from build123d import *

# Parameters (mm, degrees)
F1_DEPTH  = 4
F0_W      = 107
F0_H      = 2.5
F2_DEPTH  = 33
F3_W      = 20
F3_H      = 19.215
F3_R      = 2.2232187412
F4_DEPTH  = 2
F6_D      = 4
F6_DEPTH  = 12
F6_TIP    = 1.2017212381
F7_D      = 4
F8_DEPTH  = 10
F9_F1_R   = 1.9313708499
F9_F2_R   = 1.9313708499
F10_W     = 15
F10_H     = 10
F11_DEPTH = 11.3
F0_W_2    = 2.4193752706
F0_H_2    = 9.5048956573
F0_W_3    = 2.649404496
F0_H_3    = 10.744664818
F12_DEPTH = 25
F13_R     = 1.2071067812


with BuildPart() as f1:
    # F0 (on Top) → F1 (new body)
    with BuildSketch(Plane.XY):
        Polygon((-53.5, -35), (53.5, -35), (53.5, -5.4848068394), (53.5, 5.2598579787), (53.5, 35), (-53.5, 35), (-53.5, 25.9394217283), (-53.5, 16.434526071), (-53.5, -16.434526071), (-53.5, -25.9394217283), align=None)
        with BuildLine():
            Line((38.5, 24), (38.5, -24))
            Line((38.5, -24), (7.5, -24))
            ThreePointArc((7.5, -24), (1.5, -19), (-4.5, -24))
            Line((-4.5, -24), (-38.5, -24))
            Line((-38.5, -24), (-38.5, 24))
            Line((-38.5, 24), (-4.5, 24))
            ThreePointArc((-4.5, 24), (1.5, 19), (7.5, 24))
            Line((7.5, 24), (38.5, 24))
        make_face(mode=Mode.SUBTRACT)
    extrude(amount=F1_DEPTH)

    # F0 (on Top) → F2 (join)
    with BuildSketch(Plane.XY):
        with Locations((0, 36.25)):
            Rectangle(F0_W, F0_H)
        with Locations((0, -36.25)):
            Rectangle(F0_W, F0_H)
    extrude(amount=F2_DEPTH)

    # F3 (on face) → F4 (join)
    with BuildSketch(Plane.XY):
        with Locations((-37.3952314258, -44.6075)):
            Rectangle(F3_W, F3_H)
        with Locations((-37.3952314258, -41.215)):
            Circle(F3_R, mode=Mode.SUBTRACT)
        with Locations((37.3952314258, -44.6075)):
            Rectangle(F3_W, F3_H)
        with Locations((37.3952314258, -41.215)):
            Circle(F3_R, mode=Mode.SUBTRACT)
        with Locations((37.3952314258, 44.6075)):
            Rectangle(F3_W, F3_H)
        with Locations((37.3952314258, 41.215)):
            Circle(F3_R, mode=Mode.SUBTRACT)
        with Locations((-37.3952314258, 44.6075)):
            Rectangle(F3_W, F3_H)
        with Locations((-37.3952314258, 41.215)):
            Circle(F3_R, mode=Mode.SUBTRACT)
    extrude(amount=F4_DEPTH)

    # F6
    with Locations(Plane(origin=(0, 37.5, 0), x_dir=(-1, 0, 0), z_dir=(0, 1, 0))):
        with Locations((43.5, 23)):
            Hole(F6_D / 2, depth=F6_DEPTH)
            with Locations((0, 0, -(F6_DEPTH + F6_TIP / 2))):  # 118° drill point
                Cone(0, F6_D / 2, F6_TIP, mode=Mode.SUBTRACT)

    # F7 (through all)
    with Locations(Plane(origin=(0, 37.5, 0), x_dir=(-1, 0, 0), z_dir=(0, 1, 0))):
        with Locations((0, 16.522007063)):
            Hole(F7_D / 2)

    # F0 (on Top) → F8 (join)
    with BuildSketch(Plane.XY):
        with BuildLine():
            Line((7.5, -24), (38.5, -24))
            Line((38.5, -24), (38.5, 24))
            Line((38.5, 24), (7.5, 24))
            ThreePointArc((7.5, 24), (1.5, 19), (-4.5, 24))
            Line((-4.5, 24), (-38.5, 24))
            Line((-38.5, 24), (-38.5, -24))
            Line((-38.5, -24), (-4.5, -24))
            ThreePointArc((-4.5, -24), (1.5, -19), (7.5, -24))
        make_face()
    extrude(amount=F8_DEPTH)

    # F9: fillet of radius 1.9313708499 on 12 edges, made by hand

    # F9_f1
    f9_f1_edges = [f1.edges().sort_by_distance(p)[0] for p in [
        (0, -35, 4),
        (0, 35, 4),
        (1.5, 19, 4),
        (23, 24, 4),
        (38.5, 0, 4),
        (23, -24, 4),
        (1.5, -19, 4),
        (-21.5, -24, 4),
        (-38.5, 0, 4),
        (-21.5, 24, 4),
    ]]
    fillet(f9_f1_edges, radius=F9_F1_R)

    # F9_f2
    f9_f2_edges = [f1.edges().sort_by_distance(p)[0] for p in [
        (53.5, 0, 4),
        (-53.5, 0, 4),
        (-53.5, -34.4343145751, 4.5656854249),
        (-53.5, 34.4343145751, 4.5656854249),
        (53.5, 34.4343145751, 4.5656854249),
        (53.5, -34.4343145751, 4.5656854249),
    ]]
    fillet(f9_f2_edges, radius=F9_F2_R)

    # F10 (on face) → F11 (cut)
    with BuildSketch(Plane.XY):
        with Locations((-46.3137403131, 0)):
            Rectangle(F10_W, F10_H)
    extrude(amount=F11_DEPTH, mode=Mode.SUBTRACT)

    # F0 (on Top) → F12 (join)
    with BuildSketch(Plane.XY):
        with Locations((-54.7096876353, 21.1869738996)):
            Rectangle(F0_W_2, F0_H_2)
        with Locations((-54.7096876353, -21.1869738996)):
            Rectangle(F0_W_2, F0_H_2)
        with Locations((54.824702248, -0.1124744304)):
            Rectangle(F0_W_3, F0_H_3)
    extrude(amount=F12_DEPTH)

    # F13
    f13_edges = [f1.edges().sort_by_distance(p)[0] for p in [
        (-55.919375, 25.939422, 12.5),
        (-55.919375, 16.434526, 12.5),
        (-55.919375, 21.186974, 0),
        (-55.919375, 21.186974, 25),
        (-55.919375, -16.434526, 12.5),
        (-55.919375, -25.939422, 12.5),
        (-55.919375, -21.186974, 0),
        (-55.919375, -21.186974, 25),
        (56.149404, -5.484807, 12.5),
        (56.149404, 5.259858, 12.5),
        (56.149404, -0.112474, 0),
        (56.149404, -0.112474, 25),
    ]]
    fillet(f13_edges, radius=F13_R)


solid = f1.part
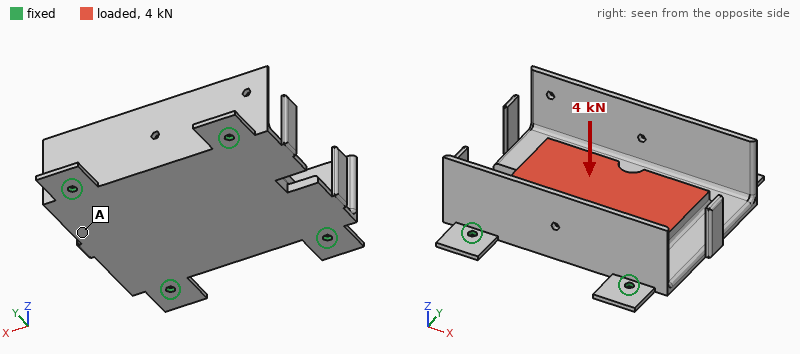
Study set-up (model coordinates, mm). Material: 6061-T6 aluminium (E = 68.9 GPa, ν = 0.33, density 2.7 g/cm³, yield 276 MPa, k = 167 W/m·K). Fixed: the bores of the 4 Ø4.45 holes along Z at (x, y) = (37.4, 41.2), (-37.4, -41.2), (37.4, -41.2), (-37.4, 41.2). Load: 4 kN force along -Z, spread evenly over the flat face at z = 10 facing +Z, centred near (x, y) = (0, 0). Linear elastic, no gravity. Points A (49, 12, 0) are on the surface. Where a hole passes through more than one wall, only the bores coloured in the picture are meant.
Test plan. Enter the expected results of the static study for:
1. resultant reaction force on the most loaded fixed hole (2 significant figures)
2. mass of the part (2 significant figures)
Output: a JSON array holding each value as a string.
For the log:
["1.9 kN", "200 g"]
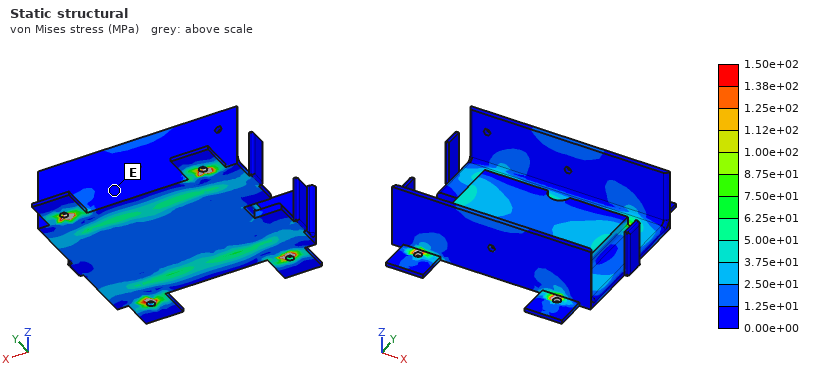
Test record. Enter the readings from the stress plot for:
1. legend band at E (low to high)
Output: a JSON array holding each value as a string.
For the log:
["0.00e+00 to 1.25e+01 MPa"]
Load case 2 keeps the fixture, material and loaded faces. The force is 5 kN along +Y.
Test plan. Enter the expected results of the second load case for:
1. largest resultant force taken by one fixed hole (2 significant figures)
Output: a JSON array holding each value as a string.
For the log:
["1.3 kN"]
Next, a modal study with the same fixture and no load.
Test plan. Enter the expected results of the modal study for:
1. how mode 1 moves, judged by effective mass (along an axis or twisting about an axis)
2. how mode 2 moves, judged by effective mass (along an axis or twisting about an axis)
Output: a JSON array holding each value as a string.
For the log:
["along Z", "along Y"]
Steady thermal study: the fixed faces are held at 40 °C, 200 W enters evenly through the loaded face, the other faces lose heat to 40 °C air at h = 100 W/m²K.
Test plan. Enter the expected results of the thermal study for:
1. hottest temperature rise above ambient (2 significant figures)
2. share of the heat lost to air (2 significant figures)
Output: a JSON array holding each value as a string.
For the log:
["56 K", "49 %"]
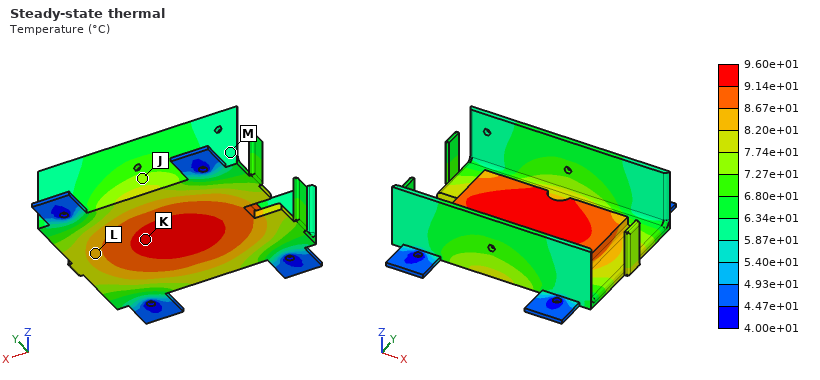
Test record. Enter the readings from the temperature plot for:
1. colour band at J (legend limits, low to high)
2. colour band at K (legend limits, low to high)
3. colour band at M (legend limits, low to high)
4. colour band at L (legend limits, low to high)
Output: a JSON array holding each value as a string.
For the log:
["7.27e+01 to 7.74e+01 °C", "9.14e+01 to 9.60e+01 °C", "5.87e+01 to 6.34e+01 °C", "8.20e+01 to 8.67e+01 °C"]
